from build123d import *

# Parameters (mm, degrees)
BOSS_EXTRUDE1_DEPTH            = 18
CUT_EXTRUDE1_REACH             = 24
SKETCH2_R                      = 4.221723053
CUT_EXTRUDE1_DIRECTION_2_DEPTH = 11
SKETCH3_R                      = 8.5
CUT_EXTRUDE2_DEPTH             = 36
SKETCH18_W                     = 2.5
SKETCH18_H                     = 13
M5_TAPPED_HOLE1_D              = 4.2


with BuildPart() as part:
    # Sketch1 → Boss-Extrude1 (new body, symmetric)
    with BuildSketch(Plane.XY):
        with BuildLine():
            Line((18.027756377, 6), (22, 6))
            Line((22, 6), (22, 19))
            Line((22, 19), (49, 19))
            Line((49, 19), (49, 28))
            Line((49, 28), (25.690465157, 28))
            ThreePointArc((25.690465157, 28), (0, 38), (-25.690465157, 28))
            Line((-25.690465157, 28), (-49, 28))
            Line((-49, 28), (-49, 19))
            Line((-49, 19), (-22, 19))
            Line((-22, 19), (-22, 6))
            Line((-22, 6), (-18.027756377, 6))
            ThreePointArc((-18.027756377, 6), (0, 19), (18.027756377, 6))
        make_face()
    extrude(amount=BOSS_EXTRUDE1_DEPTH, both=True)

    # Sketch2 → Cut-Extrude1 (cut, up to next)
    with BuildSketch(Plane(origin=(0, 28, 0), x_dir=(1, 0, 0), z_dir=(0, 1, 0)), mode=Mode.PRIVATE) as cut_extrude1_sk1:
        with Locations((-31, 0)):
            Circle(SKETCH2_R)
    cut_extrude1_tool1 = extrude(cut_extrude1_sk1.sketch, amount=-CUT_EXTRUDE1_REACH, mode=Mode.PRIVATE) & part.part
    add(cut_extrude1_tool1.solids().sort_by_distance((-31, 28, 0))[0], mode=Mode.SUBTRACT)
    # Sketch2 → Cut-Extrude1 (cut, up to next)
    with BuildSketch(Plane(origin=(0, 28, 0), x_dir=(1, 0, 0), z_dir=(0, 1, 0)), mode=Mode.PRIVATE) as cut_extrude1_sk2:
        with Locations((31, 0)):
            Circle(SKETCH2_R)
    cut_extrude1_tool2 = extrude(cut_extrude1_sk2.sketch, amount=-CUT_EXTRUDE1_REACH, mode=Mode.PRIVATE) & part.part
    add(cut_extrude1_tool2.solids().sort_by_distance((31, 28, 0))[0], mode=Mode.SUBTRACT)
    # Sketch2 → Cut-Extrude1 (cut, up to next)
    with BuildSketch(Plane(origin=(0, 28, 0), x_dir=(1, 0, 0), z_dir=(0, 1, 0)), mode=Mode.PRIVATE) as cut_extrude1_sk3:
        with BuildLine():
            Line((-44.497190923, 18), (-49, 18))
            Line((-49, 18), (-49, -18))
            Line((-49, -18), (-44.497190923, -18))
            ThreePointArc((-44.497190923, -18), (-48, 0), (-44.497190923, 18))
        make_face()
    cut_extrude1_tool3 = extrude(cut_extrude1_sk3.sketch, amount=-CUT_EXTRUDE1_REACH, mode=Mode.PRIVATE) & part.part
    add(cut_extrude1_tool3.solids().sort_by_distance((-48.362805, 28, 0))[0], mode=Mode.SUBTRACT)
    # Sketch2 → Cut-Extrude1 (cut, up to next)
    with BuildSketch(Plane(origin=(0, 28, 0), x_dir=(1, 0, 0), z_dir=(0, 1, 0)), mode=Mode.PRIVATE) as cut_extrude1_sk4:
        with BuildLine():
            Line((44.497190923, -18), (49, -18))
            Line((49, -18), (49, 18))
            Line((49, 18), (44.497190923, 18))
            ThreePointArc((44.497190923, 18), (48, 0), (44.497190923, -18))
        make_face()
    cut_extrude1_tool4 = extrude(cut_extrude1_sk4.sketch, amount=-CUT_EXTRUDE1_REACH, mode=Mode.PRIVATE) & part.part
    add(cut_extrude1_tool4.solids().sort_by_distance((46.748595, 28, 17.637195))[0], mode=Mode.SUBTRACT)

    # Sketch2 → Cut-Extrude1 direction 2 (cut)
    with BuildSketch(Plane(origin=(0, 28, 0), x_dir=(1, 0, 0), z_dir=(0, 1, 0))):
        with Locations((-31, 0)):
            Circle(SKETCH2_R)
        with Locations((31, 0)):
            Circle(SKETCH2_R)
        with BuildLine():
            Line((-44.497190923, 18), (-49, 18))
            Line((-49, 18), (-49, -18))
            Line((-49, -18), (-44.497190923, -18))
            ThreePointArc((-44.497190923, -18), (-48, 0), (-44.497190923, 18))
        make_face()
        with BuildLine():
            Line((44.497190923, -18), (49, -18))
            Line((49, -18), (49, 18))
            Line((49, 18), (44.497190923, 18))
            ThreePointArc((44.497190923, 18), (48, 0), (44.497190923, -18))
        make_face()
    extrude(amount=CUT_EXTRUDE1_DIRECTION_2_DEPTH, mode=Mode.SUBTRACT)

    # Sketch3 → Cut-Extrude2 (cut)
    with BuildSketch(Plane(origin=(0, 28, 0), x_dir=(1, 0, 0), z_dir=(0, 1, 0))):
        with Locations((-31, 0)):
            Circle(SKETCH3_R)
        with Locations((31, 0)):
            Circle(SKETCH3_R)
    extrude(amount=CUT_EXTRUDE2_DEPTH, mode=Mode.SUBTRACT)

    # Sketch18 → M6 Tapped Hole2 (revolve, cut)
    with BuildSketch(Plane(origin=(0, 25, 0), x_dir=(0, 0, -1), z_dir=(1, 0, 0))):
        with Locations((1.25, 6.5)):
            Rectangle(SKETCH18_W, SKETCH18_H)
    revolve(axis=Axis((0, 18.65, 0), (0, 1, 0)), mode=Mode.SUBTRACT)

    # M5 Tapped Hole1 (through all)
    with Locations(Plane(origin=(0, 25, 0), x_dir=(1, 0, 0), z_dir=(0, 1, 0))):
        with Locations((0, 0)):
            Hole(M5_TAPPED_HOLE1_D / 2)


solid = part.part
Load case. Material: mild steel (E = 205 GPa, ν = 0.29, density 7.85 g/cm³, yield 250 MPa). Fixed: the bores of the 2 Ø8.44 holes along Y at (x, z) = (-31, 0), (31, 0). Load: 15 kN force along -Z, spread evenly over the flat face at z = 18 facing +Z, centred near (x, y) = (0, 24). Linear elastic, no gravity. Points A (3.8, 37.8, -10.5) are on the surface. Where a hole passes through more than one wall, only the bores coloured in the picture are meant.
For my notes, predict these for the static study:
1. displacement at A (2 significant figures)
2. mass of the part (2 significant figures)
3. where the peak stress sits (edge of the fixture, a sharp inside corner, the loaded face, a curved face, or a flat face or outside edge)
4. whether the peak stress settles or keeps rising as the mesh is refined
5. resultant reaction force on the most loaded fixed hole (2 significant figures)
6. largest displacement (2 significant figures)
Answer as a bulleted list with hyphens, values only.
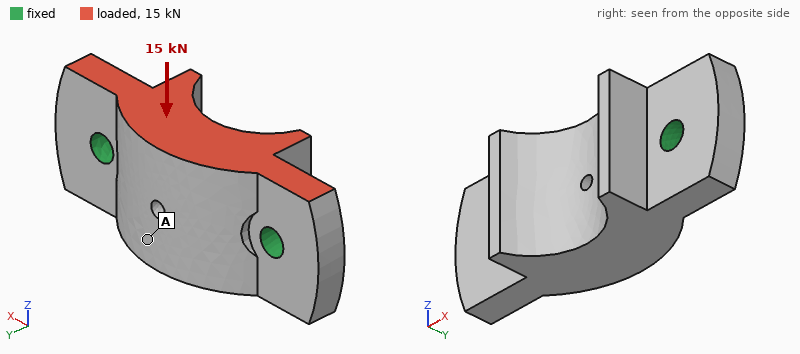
- 6.3 µm
- 390 g
- edge of the fixture
- keeps rising
- 7.5 kN
- 7.8 µm
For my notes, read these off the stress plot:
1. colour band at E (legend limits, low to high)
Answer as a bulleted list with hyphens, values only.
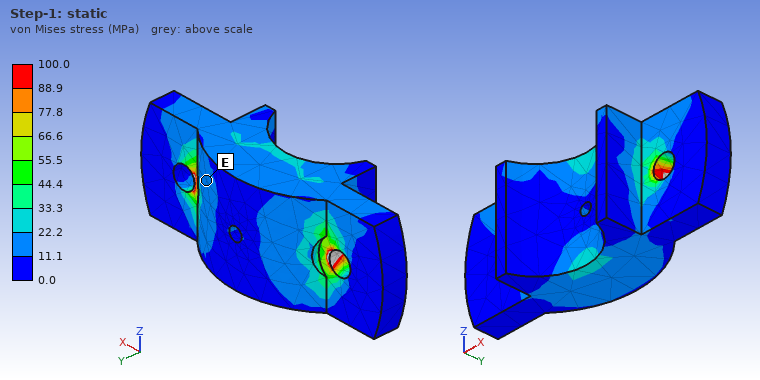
- 11.1 to 22.2 MPa
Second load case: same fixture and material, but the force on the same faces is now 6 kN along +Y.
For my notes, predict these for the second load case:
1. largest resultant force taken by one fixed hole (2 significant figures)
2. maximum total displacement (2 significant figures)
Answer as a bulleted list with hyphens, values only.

- 3.1 kN
- 19 µm
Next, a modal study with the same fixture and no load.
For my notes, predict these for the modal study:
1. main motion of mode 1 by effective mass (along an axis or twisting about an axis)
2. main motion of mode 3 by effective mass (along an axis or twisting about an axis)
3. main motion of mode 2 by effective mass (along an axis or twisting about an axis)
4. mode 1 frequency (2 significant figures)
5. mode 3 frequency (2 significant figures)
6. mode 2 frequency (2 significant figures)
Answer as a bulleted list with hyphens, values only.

- twisting about X
- along Z
- along Y
- 8800 Hz
- 15 kHz
- 11 kHz
